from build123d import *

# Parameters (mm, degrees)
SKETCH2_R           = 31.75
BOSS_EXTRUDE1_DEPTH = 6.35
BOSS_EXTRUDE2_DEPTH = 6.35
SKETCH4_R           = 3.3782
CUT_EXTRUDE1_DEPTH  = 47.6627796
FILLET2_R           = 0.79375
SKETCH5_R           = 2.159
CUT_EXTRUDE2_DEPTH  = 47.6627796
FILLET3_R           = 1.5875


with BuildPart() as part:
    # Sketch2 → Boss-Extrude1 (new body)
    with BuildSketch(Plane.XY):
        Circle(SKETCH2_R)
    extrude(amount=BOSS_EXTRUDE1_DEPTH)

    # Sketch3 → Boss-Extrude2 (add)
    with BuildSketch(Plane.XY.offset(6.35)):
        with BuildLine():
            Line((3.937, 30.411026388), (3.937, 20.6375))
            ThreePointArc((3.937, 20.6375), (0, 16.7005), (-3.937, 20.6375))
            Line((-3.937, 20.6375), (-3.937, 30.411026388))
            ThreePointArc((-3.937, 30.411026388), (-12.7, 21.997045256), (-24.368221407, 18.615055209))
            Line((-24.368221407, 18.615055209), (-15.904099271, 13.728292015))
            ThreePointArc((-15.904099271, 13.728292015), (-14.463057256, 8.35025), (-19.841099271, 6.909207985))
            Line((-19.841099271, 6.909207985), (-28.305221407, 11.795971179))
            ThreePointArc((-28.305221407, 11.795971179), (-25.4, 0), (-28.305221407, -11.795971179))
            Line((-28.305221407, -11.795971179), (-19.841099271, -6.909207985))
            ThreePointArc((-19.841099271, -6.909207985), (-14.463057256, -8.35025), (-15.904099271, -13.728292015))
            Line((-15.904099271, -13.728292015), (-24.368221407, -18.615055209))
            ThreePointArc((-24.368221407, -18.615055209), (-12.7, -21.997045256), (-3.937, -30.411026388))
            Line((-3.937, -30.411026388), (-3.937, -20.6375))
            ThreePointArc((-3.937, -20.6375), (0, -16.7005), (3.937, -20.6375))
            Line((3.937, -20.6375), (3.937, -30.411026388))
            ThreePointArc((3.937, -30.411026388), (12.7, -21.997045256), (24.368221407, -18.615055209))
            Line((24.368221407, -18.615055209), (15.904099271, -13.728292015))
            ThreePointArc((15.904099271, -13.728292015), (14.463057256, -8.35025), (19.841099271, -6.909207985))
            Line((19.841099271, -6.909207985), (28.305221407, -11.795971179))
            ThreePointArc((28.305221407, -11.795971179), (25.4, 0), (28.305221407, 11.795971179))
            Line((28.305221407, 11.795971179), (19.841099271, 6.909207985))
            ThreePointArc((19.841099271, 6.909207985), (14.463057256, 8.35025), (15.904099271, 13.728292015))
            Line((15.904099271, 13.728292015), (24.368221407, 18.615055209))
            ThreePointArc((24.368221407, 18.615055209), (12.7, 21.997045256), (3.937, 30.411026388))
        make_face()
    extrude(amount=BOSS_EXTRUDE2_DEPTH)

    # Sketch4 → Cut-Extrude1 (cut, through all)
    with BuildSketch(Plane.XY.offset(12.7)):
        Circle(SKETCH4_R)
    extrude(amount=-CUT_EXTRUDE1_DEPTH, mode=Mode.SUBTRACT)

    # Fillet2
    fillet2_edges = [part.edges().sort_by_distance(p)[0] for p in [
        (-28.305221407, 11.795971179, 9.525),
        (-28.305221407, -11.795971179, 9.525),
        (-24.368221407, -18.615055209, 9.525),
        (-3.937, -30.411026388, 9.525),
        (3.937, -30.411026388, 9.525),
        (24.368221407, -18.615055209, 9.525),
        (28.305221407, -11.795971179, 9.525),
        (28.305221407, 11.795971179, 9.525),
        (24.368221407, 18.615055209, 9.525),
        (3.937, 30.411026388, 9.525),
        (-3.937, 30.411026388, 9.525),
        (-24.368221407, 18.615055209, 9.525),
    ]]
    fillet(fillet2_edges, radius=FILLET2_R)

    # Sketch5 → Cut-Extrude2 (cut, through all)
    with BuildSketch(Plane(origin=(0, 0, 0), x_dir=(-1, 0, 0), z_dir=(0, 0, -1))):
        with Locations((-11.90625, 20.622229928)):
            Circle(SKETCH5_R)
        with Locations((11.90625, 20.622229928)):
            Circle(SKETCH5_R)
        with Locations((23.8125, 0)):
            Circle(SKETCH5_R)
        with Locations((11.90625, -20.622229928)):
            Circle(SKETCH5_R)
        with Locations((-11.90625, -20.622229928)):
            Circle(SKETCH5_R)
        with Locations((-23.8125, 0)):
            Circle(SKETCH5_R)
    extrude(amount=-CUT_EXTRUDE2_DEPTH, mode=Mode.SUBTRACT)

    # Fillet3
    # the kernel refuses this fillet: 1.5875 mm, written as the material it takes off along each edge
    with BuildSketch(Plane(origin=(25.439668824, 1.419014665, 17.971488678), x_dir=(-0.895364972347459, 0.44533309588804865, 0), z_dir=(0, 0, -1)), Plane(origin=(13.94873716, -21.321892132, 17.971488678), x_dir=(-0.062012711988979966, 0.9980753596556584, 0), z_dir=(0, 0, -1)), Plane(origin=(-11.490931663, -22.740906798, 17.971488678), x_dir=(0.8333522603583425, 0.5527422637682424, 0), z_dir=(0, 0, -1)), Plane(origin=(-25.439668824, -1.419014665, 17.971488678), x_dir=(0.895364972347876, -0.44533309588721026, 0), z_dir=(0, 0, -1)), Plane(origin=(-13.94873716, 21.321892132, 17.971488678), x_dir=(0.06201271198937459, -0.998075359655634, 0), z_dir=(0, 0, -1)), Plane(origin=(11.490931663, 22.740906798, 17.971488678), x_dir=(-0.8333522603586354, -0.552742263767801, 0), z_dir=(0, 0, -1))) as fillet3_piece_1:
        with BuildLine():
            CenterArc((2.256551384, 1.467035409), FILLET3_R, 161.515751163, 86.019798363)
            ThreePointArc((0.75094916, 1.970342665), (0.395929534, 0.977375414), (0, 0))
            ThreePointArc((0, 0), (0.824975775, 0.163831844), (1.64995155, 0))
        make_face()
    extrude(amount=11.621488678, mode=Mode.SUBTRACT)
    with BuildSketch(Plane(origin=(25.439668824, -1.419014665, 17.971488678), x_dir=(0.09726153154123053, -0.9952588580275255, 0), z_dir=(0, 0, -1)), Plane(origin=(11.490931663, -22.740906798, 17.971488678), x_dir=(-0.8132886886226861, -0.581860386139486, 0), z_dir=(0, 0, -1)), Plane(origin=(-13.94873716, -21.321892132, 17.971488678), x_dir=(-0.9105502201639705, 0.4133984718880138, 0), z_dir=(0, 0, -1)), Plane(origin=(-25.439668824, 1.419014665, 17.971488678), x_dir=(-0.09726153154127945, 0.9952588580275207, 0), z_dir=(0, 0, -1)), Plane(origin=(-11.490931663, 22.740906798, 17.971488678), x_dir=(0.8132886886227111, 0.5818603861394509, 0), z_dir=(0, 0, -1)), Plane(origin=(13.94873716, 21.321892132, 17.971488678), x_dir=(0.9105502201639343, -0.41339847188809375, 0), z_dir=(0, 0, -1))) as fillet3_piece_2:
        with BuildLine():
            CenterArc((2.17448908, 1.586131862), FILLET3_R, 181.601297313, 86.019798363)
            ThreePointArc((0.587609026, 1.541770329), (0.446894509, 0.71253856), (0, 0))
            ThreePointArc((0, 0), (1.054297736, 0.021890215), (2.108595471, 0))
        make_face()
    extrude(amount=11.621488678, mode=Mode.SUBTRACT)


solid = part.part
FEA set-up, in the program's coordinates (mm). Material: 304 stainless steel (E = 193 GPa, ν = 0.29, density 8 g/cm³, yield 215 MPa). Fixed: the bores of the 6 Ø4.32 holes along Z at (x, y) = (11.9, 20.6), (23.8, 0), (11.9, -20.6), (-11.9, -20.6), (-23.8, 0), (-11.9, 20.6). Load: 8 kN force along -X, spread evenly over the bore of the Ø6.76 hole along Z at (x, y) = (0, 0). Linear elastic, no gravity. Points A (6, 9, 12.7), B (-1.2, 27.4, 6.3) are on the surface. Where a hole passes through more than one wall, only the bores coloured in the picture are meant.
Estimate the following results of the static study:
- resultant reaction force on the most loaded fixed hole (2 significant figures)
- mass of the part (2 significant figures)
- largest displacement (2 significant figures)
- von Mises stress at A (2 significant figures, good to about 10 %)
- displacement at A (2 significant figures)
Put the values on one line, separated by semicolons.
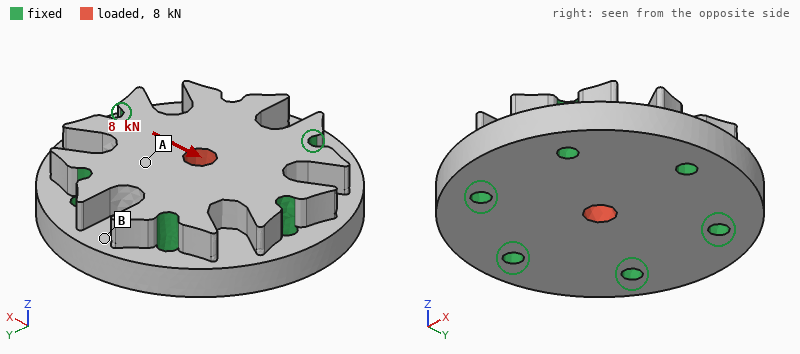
2.2 kN; 240 g; 1.9 µm; 10 MPa; 0.81 µm
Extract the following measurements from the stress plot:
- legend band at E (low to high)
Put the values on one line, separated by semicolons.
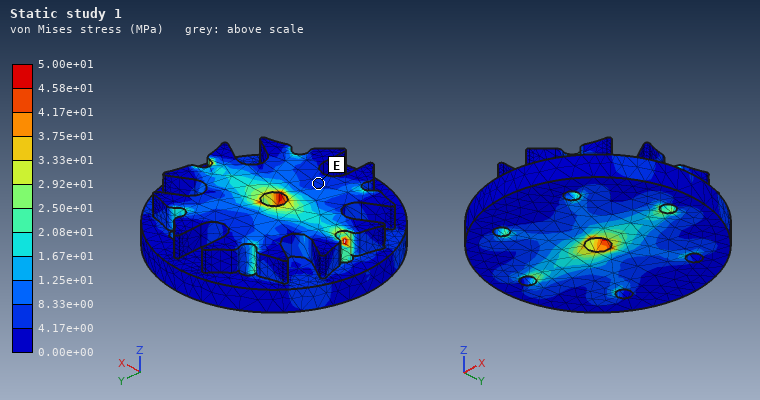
4.17e+00 to 8.33e+00 MPa
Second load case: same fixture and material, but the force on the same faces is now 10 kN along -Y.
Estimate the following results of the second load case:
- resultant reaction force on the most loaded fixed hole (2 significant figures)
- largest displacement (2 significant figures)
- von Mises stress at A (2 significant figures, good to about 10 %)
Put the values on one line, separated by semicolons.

2.4 kN; 2.4 µm; 20 MPa
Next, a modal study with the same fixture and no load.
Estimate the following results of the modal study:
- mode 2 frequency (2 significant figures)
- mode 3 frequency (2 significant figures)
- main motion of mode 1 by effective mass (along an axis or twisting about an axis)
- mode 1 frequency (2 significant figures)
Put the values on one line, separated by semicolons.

42 kHz; 43 kHz; along Z; 30 kHz
